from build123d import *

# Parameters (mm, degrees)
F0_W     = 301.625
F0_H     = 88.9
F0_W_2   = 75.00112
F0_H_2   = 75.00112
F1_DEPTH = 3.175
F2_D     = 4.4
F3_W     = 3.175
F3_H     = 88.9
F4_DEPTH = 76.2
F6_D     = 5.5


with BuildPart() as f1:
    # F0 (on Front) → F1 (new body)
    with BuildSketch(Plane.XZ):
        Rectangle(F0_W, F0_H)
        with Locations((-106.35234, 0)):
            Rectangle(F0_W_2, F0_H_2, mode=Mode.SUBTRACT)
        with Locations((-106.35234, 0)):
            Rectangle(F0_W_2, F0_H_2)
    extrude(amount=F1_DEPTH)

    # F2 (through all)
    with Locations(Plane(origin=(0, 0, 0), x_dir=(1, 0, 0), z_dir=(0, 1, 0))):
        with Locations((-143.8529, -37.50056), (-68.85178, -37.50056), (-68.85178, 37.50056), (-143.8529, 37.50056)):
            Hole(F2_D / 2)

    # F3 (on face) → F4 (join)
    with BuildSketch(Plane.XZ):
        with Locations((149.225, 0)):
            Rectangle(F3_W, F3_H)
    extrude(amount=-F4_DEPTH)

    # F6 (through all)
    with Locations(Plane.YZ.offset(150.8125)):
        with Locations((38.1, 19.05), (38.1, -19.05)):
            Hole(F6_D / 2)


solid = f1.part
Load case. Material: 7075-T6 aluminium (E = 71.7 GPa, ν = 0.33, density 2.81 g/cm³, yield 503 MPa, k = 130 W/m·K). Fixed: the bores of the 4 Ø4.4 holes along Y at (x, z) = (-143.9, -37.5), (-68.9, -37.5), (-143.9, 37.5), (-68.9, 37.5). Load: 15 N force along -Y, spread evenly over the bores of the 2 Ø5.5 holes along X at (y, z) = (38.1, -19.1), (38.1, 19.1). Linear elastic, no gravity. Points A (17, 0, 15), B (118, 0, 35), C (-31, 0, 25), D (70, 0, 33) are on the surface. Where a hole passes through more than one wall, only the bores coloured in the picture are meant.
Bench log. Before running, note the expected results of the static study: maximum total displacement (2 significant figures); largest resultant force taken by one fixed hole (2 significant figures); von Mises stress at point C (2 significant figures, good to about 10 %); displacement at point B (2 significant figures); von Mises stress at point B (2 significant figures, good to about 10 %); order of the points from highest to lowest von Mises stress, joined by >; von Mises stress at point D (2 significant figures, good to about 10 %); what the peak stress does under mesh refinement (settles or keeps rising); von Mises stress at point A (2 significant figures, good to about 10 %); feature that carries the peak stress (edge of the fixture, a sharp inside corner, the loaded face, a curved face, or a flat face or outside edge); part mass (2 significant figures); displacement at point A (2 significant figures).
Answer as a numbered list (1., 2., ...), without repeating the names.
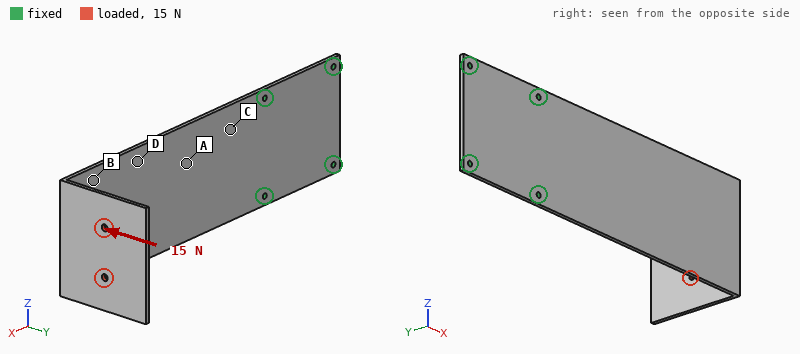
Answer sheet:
1. 3.6 mm
2. 15 N
3. 17 MPa
4. 2.5 mm
5. 3.4 MPa
6. C > A > D > B
7. 8.1 MPa
8. keeps rising
9. 13 MPa
10. edge of the fixture
11. 300 g
12. 0.69 mm
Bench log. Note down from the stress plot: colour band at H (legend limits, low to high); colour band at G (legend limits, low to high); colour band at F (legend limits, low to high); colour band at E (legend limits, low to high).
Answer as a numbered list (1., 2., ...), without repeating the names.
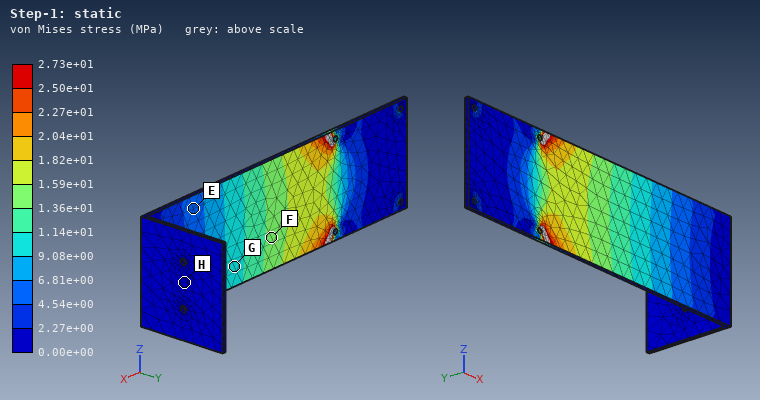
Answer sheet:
1. 0.00e+00 to 2.27e+00 MPa
2. 9.08e+00 to 1.14e+01 MPa
3. 1.36e+01 to 1.59e+01 MPa
4. 4.54e+00 to 6.81e+00 MPa
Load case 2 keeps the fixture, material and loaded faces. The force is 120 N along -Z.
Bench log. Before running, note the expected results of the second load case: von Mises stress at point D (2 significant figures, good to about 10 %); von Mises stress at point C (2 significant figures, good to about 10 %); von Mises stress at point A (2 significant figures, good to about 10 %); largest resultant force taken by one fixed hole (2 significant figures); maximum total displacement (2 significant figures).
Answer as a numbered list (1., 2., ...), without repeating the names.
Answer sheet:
1. 28 MPa
2. 24 MPa
3. 28 MPa
4. 330 N
5. 3.2 mm
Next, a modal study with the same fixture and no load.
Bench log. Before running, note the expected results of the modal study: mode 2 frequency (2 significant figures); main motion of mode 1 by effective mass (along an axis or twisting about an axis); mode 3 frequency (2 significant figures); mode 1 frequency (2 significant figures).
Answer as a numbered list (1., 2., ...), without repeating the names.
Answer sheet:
1. 130 Hz
2. along Y
3. 180 Hz
4. 33 Hz
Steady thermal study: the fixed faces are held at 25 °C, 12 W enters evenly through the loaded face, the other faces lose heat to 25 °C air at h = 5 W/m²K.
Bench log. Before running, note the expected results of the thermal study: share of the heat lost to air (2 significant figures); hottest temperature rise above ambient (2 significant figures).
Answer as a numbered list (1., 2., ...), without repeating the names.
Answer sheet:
1. 59 %
2. 51 K
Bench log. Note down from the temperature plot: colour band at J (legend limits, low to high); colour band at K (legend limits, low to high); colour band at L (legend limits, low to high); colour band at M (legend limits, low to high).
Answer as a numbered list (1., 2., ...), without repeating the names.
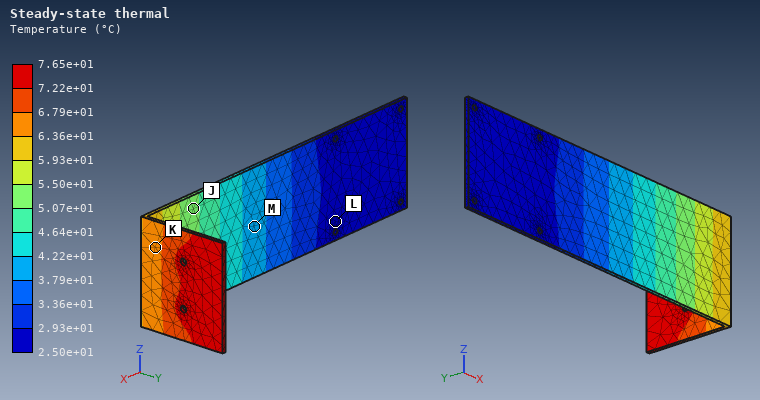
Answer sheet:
1. 5.07e+01 to 5.50e+01 °C
2. 6.36e+01 to 6.79e+01 °C
3. 2.50e+01 to 2.93e+01 °C
4. 3.79e+01 to 4.22e+01 °C
